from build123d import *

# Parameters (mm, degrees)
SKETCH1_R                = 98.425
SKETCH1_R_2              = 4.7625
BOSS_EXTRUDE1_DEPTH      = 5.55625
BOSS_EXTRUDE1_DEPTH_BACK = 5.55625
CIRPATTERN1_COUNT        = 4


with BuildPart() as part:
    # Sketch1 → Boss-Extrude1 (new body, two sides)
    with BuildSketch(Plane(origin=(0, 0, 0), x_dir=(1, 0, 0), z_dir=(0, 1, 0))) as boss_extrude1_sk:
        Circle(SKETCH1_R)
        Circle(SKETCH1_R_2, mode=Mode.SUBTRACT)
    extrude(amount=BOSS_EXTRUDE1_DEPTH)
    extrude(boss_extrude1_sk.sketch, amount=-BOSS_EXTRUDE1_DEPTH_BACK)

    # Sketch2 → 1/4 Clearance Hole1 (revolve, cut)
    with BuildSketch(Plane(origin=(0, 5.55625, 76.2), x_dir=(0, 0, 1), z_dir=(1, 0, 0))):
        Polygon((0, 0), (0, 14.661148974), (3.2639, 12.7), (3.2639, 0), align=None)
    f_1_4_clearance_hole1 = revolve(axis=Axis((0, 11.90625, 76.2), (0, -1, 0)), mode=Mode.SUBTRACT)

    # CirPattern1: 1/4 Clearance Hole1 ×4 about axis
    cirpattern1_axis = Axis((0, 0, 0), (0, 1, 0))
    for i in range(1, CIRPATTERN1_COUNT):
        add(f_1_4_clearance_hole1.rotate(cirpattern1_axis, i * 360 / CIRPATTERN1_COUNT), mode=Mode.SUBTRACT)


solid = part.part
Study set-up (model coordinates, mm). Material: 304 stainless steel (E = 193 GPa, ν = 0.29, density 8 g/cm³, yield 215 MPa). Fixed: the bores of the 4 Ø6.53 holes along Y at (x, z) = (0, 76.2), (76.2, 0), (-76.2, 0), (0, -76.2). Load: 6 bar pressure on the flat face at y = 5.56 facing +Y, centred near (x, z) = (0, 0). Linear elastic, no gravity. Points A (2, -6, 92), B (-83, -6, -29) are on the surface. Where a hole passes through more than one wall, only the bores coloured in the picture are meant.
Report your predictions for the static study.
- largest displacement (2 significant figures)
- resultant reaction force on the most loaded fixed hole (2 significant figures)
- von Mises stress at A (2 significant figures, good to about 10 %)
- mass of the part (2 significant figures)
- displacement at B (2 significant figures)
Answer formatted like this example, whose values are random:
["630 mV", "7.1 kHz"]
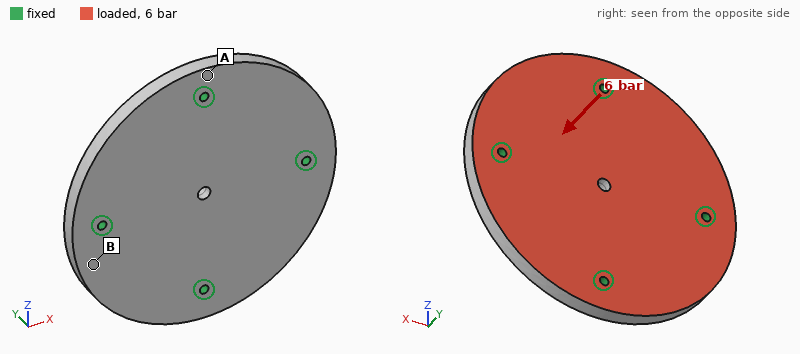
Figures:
["25 µm", "4.5 kN", "22 MPa", "2.7 kg", "8.4 µm"]
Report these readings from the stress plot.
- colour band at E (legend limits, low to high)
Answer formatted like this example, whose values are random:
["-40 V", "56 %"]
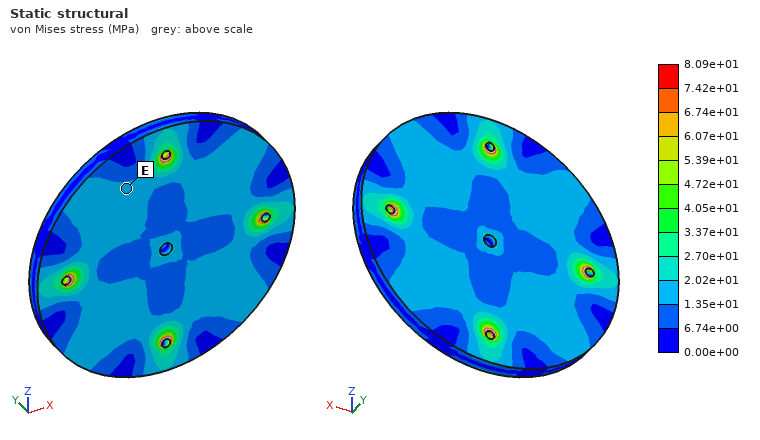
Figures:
["1.35e+01 to 2.02e+01 MPa"]
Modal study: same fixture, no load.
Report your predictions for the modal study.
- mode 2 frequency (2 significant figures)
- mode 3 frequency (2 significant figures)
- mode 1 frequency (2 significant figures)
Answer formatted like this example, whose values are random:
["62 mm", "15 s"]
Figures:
["3000 Hz", "3100 Hz", "2700 Hz"]
